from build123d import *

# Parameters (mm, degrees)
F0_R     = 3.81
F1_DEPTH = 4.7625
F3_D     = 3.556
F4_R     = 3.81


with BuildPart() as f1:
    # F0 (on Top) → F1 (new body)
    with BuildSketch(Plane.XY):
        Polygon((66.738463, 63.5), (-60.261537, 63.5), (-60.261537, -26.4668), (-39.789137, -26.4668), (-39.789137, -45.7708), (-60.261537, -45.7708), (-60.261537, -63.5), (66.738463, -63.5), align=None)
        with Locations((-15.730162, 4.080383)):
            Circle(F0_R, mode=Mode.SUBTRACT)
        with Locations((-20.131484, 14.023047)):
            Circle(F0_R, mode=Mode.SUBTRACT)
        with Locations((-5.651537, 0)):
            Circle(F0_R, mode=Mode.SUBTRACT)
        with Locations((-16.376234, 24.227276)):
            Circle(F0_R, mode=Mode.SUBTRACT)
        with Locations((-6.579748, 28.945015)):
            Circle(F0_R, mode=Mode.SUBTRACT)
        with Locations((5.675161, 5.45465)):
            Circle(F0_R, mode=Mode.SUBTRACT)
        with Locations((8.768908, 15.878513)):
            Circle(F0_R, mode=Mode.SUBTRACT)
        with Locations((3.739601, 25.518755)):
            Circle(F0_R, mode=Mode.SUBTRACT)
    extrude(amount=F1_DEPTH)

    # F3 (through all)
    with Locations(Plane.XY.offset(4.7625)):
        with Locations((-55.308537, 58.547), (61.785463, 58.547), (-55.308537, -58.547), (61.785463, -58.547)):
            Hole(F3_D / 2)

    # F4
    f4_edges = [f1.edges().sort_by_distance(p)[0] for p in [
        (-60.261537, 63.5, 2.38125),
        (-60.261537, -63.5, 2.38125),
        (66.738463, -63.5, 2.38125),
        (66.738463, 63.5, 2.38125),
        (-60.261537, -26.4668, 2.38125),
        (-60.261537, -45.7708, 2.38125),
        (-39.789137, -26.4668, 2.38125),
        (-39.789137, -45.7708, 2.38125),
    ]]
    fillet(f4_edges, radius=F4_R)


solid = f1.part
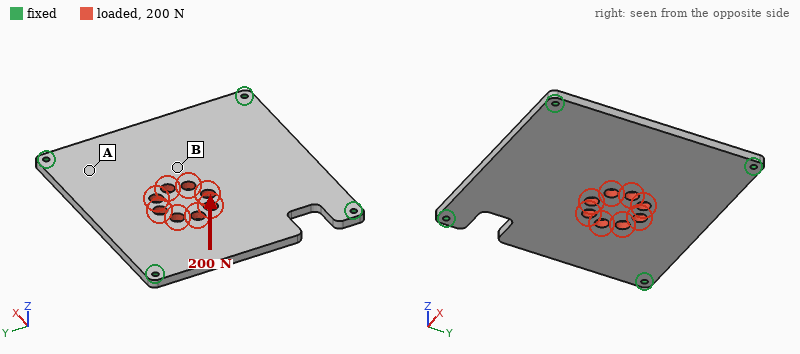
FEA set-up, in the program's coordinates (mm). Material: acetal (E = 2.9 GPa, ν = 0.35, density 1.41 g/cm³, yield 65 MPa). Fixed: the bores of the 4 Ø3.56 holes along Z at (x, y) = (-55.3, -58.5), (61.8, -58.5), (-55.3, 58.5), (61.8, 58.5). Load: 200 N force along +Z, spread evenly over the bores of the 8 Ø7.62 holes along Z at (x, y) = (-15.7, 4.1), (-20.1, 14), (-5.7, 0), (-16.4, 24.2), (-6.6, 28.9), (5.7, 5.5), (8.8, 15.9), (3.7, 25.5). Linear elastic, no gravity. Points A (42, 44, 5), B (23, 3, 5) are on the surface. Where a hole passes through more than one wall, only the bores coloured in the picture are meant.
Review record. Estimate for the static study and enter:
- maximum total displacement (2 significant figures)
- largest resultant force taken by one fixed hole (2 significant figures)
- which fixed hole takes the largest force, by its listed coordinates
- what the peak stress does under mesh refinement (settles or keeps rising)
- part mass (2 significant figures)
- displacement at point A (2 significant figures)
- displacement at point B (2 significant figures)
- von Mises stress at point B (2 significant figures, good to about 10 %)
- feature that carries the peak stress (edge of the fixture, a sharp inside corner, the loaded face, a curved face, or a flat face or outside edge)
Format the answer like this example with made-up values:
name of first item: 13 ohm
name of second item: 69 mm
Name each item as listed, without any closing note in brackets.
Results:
maximum total displacement: 1.8 mm
largest resultant force taken by one fixed hole: 79 N
which fixed hole takes the largest force, by its listed coordinates: (-55.3, 58.5)
what the peak stress does under mesh refinement: keeps rising
part mass: 100 g
displacement at point A: 0.54 mm
displacement at point B: 1.4 mm
von Mises stress at point B: 6.3 MPa
feature that carries the peak stress: edge of the fixture
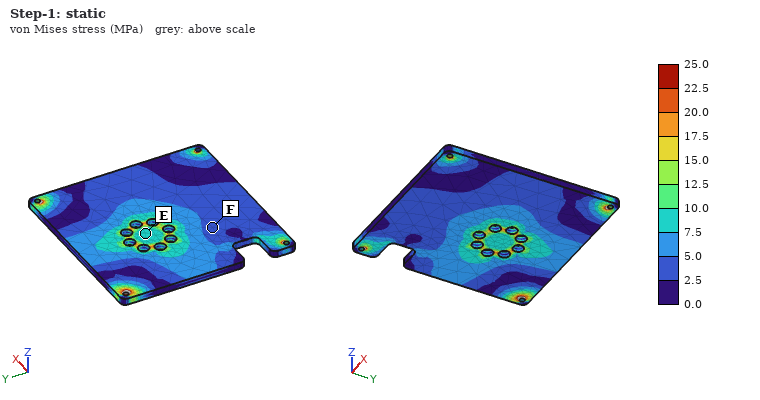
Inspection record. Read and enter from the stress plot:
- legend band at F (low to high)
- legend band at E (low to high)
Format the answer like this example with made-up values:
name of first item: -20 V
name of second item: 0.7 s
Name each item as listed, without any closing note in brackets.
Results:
legend band at F: 2.5 to 5.0 MPa
legend band at E: 7.5 to 10.0 MPa
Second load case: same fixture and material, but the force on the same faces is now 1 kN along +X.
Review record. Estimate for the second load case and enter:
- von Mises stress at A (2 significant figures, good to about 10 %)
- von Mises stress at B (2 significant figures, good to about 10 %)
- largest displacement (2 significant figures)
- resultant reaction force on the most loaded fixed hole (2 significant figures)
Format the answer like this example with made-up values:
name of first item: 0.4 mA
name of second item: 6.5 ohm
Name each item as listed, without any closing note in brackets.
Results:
von Mises stress at A: 2.5 MPa
von Mises stress at B: 1.4 MPa
largest displacement: 92 µm
resultant reaction force on the most loaded fixed hole: 350 N
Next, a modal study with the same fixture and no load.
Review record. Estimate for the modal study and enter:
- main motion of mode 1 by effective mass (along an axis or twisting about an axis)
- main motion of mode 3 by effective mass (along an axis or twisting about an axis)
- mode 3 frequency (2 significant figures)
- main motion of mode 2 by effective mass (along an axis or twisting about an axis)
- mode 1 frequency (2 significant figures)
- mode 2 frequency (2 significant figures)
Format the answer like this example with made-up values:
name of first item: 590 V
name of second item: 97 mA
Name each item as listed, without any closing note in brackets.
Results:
main motion of mode 1 by effective mass: along Z
main motion of mode 3 by effective mass: twisting about X
mode 3 frequency: 530 Hz
main motion of mode 2 by effective mass: twisting about Y
mode 1 frequency: 280 Hz
mode 2 frequency: 470 Hz
